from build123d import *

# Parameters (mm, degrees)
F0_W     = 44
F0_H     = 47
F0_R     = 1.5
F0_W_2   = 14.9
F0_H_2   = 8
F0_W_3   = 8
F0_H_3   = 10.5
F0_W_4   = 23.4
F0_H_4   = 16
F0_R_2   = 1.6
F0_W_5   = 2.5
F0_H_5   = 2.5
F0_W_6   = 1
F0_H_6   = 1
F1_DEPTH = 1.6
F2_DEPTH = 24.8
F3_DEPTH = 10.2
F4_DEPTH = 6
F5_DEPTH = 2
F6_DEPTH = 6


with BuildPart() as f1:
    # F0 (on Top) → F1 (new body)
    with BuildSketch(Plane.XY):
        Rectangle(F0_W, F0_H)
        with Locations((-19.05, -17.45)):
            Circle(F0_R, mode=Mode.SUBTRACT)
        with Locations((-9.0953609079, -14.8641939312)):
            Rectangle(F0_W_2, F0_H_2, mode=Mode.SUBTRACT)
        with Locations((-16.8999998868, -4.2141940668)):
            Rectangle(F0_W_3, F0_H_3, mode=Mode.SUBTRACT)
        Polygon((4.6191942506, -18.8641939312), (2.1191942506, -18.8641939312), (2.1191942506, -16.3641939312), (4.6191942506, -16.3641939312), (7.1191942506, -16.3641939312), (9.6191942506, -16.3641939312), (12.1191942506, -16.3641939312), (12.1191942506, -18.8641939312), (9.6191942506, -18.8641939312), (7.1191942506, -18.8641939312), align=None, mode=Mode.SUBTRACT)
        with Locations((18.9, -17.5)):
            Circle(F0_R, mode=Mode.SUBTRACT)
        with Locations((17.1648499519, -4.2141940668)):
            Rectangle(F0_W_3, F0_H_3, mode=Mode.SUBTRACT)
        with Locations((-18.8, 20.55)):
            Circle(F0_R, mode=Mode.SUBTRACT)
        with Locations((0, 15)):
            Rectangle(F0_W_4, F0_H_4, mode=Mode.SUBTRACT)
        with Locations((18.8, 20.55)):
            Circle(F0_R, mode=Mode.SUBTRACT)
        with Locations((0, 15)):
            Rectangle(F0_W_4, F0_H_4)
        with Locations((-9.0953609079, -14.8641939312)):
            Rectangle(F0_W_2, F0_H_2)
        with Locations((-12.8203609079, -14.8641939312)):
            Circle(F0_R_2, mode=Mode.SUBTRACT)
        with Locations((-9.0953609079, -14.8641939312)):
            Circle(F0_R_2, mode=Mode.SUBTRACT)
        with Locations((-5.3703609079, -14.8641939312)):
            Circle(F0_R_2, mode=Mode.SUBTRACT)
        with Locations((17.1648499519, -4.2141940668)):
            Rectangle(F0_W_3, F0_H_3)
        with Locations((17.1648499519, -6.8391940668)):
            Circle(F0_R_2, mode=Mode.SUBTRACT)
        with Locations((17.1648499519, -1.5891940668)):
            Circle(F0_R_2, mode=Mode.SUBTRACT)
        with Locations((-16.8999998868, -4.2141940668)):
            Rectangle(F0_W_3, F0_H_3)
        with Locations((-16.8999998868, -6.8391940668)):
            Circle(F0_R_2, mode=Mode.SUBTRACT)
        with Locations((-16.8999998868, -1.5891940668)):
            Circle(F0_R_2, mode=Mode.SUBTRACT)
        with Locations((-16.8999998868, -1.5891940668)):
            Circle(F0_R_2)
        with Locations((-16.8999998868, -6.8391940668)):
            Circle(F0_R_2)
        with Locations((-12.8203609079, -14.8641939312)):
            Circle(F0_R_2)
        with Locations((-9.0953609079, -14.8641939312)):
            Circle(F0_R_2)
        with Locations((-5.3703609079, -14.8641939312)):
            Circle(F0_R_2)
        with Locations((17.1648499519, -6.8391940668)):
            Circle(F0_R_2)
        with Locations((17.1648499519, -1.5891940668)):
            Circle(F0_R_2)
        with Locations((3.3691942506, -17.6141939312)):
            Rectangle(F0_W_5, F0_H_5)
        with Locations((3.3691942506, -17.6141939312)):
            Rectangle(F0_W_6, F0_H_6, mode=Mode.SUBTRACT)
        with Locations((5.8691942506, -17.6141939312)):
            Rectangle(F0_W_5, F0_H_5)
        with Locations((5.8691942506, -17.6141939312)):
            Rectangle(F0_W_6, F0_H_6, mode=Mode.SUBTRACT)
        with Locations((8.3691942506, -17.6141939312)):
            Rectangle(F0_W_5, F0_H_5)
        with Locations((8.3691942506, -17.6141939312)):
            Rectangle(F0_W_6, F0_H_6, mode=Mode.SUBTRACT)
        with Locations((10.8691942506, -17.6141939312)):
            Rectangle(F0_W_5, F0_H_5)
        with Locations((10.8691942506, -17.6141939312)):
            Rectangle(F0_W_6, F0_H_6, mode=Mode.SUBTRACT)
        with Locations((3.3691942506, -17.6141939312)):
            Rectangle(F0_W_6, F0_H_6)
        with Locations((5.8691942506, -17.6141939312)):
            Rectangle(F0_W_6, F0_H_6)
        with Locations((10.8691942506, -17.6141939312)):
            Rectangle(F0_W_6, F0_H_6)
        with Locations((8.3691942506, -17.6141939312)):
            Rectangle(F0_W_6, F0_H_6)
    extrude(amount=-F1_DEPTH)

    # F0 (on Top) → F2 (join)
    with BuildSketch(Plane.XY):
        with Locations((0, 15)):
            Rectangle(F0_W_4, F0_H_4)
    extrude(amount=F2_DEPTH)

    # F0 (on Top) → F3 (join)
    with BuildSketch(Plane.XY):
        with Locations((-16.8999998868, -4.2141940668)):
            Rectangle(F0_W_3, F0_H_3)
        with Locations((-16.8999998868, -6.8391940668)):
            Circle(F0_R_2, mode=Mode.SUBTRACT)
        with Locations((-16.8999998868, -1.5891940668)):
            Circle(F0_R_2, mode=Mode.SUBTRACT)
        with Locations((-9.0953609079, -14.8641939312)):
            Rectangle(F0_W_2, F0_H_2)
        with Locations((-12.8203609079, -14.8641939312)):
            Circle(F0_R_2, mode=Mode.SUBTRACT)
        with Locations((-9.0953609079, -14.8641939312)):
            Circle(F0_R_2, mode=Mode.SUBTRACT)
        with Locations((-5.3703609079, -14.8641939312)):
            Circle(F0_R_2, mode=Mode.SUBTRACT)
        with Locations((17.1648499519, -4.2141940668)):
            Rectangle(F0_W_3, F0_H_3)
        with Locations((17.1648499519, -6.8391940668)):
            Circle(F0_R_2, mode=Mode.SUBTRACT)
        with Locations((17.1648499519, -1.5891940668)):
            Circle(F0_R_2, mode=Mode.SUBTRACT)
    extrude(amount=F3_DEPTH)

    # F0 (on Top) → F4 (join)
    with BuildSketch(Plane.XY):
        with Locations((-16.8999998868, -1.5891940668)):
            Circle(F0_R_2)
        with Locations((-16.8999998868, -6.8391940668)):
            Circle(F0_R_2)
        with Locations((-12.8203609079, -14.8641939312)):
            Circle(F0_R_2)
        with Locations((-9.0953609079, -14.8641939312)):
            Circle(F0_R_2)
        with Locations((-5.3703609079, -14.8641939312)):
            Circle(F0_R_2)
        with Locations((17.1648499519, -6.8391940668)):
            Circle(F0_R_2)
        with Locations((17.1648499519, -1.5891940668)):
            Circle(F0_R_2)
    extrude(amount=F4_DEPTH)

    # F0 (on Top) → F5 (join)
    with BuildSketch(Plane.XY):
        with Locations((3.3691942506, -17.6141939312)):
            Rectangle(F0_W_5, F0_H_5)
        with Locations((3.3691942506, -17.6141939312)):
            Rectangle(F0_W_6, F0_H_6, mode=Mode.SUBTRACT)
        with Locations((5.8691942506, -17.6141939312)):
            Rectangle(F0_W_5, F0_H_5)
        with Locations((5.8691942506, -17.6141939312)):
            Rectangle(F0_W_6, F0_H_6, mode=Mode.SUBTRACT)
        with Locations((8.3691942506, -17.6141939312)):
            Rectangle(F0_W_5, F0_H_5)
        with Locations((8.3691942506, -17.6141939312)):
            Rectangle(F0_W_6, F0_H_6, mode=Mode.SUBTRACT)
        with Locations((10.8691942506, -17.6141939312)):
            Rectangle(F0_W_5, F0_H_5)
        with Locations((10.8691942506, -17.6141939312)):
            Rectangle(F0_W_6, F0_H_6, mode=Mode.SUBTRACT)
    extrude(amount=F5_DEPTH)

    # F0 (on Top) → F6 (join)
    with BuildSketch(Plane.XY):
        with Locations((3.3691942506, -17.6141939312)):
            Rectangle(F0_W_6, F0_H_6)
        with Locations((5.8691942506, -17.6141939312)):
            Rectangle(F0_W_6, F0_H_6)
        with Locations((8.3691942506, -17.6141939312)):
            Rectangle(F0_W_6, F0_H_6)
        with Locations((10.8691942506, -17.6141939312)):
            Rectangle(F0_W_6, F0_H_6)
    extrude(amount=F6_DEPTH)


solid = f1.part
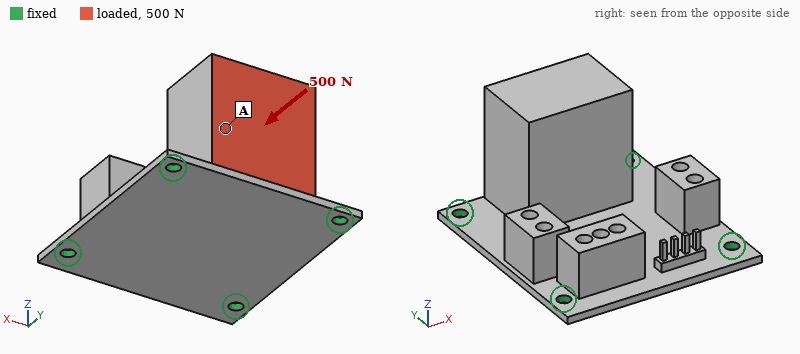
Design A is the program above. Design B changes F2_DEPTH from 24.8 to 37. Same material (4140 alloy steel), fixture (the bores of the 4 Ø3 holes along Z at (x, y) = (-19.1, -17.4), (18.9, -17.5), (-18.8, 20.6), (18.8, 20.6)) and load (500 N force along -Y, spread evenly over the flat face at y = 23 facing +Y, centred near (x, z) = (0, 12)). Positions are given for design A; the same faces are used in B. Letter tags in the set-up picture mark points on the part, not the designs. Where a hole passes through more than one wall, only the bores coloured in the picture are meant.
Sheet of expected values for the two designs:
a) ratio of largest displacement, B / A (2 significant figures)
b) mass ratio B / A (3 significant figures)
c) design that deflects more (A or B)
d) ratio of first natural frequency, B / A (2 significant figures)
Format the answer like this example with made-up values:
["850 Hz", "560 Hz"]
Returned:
["2.1", "1.30", "B", "0.60"]
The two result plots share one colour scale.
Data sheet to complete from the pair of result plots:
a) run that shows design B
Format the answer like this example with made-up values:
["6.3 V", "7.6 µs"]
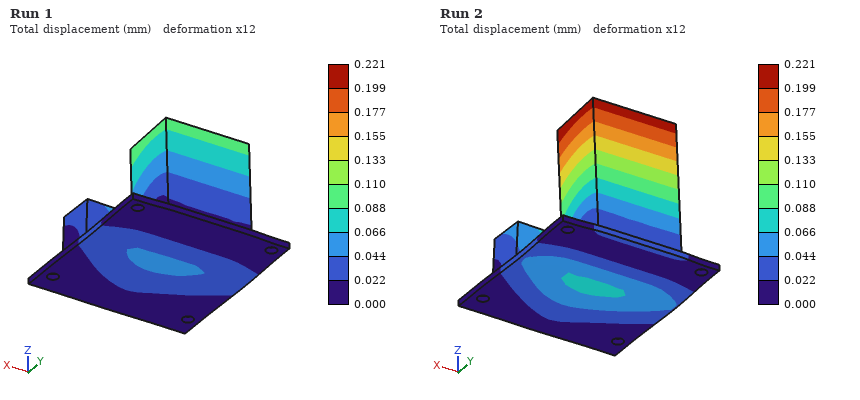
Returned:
["Run 2"]
